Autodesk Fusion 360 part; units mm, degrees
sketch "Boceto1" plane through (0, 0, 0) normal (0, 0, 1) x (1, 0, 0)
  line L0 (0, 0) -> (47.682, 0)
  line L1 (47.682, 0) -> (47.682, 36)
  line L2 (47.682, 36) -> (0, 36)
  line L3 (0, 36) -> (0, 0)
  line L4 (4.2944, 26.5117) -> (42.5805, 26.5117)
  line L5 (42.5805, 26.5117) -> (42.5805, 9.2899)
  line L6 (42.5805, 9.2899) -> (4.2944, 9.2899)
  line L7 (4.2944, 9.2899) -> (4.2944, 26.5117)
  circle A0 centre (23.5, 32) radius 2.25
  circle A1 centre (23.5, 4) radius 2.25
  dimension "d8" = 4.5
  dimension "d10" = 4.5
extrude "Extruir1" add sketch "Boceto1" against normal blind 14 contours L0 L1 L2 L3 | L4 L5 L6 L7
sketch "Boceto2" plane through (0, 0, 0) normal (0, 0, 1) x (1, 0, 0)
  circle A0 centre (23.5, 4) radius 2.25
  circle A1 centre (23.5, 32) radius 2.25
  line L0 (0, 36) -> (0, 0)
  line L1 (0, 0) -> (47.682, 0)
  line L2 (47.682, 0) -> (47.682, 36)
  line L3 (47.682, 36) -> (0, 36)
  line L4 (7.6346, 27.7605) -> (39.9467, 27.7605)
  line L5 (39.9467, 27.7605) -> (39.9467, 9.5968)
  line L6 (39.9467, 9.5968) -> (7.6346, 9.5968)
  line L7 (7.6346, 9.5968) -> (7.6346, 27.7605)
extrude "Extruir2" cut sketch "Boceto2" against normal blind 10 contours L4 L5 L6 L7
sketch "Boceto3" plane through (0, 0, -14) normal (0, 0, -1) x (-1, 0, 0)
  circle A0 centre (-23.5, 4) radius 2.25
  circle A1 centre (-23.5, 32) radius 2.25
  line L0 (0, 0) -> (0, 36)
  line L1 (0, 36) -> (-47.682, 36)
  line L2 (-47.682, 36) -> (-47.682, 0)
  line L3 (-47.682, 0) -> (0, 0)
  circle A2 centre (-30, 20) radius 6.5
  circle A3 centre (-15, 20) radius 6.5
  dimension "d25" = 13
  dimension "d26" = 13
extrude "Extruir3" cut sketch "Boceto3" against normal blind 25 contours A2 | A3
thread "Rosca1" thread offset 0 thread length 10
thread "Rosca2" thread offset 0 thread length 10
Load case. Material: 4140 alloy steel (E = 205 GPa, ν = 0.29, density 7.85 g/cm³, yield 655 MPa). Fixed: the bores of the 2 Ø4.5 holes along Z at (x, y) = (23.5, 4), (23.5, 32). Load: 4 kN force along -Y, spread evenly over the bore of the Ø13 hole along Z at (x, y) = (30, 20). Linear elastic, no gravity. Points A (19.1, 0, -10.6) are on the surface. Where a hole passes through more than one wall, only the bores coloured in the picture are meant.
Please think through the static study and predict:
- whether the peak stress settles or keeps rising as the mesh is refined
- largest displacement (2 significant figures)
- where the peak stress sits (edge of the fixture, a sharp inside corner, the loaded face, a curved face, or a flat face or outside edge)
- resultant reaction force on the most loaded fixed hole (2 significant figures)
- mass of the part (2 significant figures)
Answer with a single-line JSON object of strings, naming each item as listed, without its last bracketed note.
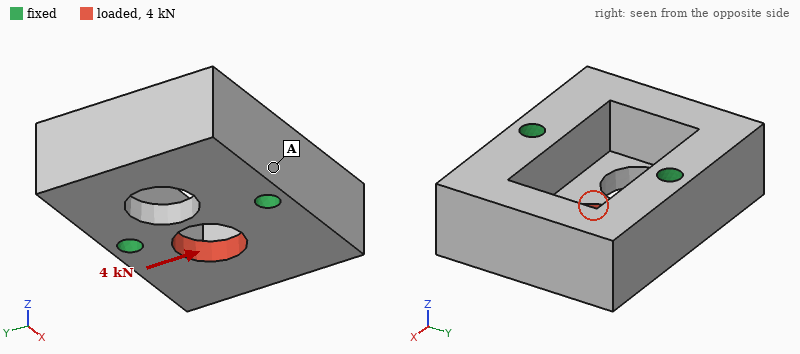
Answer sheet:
{"whether the peak stress settles or keeps rising as the mesh is refined": "keeps rising", "largest displacement": "4.7 µm", "where the peak stress sits": "edge of the fixture", "resultant reaction force on the most loaded fixed hole": "2.1 kN", "mass of the part": "130 g"}
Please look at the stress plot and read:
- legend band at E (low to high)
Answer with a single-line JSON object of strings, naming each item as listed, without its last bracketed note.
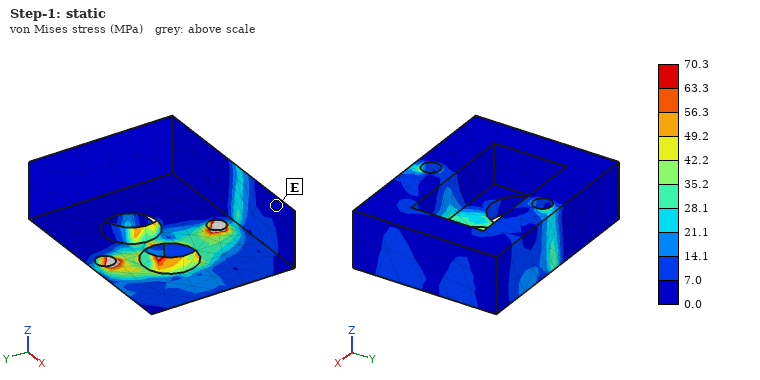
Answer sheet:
{"legend band at E": "0.0 to 7.0 MPa"}
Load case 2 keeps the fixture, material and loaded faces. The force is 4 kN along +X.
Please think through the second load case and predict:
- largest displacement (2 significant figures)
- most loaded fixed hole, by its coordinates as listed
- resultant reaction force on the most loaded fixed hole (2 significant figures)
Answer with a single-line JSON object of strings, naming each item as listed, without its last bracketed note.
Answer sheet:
{"largest displacement": "5.1 µm", "most loaded fixed hole, by its coordinates as listed": "(23.5, 32)", "resultant reaction force on the most loaded fixed hole": "2.2 kN"}
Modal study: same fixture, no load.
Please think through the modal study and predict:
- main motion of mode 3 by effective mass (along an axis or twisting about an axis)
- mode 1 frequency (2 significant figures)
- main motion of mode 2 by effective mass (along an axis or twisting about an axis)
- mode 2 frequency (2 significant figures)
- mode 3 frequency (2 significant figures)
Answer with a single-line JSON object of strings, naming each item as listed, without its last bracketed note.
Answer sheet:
{"main motion of mode 3 by effective mass": "twisting about Z", "mode 1 frequency": "13 kHz", "main motion of mode 2 by effective mass": "along Z", "mode 2 frequency": "14 kHz", "mode 3 frequency": "15 kHz"}
